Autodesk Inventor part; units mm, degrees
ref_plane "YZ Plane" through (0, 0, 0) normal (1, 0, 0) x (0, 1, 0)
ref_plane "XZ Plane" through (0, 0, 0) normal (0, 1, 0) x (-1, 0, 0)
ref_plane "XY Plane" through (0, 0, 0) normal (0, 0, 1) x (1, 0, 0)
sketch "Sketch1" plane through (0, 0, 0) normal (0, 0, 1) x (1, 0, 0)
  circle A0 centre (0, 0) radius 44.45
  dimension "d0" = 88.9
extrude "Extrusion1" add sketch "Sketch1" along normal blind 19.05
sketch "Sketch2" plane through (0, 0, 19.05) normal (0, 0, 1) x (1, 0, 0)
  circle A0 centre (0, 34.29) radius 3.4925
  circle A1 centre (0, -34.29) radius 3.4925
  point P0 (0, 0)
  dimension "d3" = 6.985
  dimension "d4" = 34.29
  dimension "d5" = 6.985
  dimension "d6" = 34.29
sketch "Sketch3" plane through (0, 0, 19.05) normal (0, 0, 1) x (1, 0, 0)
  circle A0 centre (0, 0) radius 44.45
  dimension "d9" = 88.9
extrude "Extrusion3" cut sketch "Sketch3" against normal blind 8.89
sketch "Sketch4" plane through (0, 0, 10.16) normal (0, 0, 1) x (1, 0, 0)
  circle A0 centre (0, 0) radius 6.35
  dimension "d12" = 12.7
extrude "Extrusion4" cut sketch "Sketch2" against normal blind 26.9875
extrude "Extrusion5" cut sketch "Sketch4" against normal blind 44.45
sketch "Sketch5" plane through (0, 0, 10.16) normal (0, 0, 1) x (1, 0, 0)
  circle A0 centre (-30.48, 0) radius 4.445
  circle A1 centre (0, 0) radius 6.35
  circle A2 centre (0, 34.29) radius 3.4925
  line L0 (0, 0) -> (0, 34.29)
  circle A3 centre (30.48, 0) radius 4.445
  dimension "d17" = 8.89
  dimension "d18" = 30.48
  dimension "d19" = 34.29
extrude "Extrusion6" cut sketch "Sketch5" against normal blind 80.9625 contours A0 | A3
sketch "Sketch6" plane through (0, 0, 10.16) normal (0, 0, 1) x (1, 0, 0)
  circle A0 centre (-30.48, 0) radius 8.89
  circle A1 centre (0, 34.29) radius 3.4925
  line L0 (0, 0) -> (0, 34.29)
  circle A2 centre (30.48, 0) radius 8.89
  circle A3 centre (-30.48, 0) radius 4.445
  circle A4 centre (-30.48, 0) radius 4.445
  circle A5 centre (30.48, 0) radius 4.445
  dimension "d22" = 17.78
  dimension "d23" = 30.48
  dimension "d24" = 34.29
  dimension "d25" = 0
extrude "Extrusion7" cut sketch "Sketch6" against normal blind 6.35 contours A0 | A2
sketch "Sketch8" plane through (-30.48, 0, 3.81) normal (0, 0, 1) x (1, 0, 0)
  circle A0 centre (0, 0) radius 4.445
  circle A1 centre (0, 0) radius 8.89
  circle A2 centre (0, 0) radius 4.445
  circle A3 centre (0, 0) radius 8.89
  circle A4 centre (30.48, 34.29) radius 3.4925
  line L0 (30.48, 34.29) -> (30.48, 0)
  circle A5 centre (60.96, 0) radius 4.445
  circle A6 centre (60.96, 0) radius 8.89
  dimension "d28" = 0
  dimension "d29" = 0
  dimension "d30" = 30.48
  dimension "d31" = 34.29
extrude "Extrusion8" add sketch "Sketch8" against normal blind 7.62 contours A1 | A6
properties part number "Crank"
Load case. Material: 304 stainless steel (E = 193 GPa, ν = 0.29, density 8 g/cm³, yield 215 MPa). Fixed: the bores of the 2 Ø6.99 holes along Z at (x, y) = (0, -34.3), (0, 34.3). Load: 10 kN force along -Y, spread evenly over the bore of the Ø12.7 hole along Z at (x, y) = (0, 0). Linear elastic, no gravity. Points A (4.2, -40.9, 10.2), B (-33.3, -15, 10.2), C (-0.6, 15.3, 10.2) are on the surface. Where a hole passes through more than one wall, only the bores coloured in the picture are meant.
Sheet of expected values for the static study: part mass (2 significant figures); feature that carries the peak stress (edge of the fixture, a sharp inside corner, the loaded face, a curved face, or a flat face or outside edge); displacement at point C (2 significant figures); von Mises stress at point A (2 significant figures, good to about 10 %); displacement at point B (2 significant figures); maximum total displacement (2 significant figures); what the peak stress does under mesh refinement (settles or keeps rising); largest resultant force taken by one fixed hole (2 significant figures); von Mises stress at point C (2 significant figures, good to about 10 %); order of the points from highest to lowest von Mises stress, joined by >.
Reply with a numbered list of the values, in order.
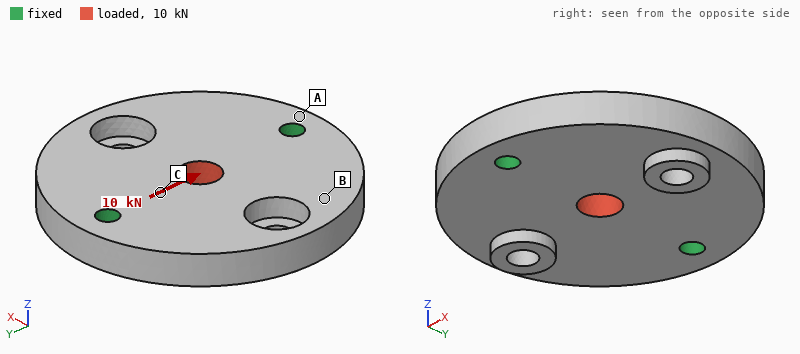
1. 470 g
2. edge of the fixture
3. 2.2 µm
4. 9.8 MPa
5. 1.9 µm
6. 3.6 µm
7. keeps rising
8. 5.0 kN
9. 25 MPa
10. C > A > B
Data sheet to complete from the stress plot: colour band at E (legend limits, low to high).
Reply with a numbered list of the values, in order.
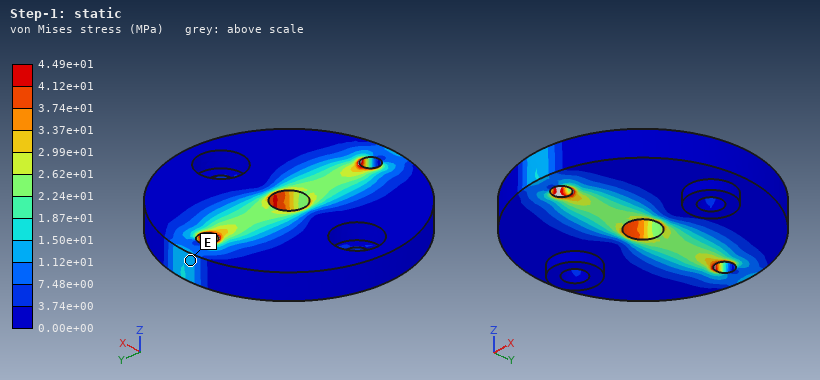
1. 1.12e+01 to 1.50e+01 MPa
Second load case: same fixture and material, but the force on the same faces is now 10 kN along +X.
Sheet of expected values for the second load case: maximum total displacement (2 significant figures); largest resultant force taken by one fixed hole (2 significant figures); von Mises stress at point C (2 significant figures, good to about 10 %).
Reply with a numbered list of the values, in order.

1. 5.8 µm
2. 5.0 kN
3. 12 MPa
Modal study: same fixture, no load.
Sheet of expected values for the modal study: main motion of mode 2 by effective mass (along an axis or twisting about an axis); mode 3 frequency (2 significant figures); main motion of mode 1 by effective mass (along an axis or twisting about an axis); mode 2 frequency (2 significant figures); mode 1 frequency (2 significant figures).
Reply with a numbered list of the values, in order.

1. along Z
2. 9100 Hz
3. twisting about Y
4. 4600 Hz
5. 3600 Hz
